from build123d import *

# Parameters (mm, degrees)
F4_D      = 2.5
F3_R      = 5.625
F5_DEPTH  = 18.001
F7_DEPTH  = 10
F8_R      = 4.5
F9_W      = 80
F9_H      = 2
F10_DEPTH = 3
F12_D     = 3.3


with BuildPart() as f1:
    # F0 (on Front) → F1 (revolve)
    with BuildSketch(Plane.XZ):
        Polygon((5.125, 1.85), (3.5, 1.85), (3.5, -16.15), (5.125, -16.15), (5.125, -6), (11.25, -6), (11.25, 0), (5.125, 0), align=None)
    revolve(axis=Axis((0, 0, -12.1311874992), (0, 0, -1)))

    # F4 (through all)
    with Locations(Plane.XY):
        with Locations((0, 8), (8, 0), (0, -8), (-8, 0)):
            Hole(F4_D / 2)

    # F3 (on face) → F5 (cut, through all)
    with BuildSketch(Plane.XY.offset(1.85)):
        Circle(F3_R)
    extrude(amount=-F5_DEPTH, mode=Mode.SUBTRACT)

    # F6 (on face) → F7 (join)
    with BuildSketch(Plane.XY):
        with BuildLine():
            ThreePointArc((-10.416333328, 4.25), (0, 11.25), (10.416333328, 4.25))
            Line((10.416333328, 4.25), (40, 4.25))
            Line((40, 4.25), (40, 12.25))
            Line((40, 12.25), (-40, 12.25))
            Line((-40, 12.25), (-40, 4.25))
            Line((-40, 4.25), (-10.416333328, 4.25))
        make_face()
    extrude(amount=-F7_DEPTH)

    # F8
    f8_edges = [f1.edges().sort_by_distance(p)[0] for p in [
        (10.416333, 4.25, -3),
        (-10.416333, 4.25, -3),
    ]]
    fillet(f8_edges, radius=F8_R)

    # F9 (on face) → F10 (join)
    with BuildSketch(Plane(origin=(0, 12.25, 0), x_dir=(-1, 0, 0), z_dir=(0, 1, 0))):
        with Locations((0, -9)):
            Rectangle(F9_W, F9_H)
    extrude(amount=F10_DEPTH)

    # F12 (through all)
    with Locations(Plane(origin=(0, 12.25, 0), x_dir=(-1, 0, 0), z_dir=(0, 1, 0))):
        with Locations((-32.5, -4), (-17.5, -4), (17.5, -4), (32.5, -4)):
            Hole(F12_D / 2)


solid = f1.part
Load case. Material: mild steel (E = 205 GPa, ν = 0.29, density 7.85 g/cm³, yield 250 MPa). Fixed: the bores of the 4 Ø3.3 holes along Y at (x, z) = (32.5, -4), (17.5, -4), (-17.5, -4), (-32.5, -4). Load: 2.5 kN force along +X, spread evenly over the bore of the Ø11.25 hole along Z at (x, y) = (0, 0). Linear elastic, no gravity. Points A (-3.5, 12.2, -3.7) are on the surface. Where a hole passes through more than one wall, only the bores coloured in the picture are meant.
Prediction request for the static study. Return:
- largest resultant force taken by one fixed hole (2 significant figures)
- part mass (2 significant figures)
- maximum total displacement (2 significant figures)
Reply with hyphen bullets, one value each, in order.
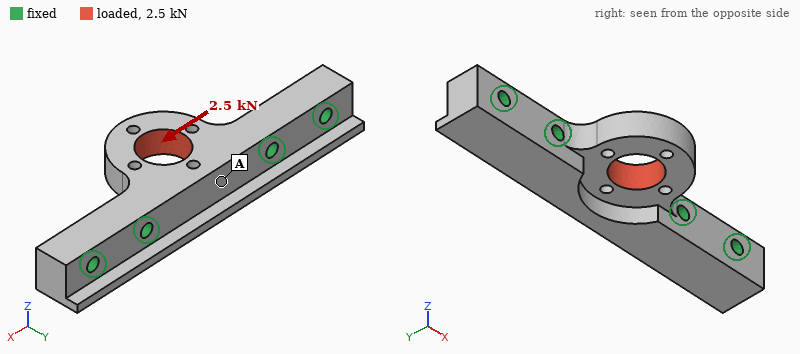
- 1.3 kN
- 57 g
- 8.8 µm
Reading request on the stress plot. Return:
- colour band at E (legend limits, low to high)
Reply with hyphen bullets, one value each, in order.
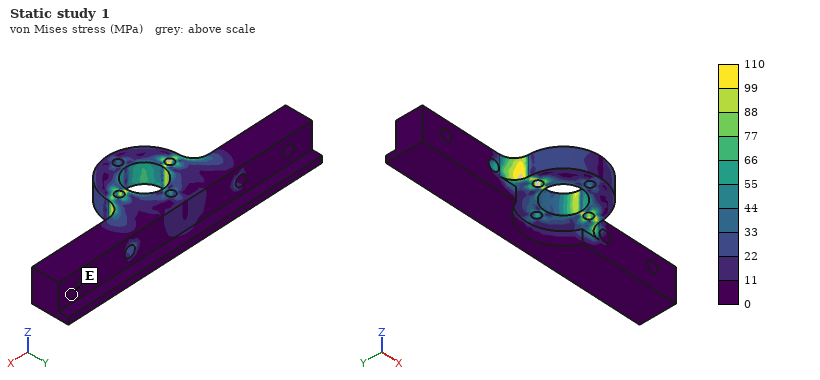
- 0 to 11 MPa
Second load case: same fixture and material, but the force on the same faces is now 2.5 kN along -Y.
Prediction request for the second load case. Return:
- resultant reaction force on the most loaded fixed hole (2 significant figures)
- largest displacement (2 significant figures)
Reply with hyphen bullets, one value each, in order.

- 1.3 kN
- 6.7 µm
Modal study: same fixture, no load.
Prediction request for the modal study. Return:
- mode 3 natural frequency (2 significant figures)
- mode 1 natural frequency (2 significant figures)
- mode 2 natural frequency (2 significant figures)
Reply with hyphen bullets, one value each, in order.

- 26 kHz
- 11 kHz
- 25 kHz
